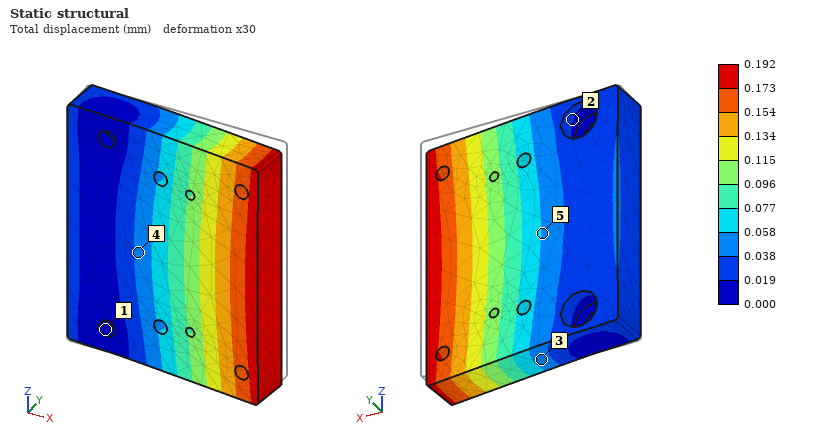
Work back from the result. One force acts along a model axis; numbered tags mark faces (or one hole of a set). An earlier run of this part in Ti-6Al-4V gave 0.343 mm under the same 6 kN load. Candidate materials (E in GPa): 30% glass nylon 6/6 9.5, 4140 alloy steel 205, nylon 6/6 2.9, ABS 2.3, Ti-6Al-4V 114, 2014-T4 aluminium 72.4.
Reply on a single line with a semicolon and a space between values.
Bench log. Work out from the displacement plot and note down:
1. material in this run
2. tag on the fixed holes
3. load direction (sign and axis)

4140 alloy steel; 1; -Y
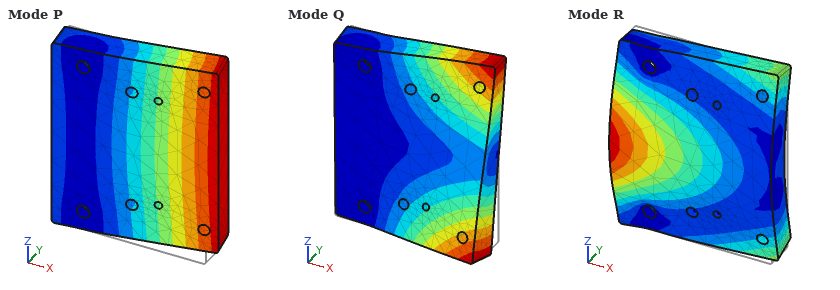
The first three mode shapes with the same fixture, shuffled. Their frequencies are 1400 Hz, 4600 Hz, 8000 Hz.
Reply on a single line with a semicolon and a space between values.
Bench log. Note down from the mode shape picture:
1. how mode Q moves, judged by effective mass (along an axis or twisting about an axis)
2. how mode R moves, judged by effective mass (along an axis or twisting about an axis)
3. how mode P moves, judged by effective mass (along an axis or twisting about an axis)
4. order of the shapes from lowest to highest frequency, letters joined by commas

twisting about X; along Y; along Y; P, Q, R
